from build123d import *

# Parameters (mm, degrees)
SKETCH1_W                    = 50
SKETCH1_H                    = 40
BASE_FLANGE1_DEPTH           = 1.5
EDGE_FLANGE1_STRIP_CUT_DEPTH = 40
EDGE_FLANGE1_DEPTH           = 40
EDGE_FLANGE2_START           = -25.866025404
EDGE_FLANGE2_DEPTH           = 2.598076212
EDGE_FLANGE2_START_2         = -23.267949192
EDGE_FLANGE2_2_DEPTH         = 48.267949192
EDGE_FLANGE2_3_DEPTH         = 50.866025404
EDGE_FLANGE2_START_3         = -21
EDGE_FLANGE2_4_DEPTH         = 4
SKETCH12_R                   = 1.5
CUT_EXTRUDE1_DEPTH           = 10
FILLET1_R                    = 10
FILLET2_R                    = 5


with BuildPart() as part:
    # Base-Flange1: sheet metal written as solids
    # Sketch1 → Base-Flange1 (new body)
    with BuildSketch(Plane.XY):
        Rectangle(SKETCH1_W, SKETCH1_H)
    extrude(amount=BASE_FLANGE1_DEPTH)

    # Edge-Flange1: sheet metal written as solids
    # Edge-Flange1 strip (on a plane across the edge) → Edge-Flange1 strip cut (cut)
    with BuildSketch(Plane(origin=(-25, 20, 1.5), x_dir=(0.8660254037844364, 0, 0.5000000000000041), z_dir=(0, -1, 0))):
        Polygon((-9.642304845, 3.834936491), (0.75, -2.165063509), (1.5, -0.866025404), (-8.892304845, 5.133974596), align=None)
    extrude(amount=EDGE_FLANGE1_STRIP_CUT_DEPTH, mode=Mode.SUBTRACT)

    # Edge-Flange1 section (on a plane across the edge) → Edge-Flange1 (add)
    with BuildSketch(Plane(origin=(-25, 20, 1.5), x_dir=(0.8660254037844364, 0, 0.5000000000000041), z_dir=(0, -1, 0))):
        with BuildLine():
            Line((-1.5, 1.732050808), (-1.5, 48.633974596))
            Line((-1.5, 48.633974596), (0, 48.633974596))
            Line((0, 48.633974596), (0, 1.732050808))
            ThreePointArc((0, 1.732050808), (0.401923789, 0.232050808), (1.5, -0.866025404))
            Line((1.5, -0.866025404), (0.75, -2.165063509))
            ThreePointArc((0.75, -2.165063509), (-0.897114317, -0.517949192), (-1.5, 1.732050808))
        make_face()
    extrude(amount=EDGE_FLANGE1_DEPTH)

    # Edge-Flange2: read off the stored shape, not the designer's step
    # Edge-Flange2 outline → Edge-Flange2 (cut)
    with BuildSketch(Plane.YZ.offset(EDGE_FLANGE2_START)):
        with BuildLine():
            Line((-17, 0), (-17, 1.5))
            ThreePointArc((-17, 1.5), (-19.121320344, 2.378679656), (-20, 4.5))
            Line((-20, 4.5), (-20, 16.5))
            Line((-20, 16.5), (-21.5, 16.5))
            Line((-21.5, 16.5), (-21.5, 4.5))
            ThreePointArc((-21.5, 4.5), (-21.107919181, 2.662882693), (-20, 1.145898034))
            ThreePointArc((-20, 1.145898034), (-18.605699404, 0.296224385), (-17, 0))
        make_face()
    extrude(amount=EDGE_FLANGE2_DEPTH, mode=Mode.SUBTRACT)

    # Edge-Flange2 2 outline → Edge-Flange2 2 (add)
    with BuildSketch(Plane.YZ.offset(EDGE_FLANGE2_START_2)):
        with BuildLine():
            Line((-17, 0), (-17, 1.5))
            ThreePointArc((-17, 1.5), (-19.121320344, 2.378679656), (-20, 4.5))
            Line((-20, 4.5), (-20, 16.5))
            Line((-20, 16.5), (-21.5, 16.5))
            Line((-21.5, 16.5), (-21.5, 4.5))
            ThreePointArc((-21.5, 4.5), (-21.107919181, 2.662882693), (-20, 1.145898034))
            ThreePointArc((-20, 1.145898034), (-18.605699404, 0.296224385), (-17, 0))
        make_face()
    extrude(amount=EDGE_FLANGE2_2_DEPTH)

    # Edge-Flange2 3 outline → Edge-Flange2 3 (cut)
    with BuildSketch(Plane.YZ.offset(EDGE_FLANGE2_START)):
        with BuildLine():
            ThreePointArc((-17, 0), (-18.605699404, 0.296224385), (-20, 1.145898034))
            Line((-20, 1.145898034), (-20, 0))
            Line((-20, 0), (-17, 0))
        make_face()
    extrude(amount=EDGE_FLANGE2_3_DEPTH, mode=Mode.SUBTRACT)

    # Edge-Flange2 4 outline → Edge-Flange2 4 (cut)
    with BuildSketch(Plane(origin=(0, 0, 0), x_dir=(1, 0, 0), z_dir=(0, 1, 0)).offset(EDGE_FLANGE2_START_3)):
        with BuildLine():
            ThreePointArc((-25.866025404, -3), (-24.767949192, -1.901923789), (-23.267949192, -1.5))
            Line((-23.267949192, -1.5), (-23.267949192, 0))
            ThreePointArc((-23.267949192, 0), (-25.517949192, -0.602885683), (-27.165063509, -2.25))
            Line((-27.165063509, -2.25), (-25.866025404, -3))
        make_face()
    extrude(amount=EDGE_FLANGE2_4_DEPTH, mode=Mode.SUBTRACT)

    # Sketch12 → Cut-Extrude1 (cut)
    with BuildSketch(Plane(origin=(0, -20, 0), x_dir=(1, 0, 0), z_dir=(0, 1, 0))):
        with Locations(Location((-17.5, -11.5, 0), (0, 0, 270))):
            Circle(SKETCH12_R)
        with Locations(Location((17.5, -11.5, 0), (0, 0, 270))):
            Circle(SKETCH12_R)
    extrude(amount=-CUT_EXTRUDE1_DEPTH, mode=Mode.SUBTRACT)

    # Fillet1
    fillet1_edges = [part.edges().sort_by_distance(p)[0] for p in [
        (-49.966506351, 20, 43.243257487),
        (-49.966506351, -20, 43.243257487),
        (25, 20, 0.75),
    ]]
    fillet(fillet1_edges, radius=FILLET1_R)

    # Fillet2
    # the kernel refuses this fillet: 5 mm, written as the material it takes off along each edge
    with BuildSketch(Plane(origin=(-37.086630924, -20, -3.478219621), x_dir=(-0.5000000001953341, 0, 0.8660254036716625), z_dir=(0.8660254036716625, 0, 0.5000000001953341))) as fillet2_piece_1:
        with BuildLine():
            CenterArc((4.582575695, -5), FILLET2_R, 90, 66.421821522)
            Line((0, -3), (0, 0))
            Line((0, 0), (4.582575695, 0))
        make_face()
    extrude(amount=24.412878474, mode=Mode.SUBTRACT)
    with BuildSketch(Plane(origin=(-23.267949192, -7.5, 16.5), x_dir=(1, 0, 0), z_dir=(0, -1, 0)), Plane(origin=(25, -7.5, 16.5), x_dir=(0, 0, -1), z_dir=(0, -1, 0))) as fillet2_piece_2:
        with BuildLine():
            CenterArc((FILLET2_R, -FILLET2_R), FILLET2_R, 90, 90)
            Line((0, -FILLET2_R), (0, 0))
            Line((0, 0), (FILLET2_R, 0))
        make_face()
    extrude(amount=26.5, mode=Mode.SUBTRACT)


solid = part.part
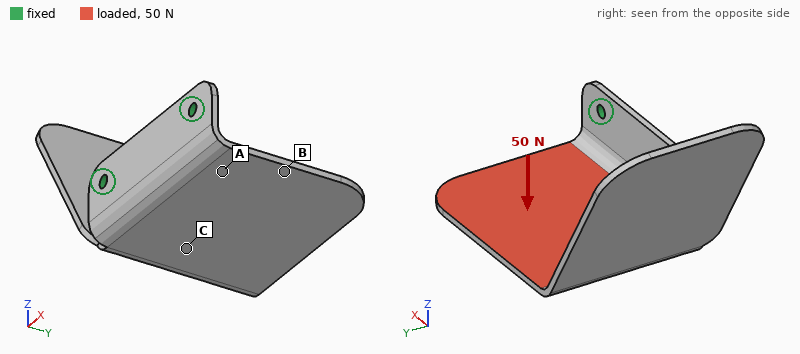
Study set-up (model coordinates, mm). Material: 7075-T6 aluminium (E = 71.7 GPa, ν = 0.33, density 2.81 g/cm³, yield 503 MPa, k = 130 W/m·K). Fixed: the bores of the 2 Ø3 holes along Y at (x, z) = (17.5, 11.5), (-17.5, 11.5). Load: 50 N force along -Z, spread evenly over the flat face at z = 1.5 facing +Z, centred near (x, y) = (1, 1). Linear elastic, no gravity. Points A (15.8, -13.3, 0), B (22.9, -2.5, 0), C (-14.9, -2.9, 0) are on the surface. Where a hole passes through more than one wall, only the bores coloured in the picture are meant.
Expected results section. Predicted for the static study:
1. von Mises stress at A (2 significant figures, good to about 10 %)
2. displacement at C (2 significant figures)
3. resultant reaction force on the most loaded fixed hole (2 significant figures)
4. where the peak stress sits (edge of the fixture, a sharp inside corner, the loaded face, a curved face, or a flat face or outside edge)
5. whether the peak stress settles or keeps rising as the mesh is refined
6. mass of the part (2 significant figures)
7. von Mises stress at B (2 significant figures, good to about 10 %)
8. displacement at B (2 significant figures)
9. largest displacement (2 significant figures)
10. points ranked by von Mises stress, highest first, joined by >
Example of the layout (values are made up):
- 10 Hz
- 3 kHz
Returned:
- 33 MPa
- 0.34 mm
- 29 N
- edge of the fixture
- keeps rising
- 19 g
- 16 MPa
- 0.32 mm
- 1.1 mm
- A > B > C
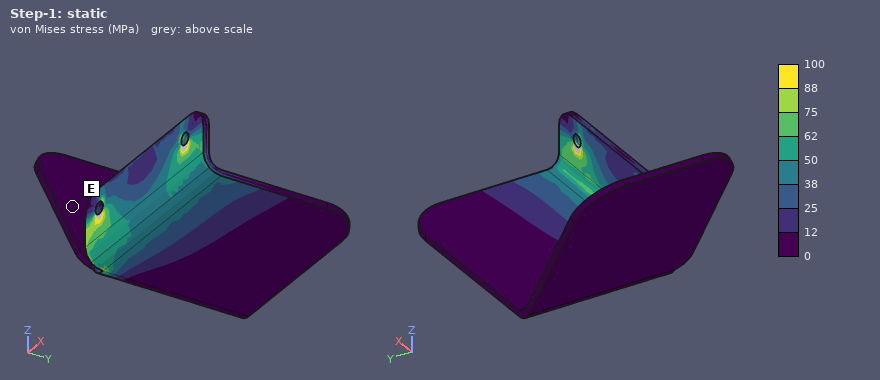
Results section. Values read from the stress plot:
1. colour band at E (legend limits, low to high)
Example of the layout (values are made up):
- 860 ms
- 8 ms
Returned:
- 0 to 12 MPa
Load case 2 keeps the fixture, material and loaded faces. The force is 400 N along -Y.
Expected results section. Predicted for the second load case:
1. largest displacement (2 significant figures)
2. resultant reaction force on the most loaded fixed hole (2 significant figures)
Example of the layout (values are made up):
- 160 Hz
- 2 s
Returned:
- 1.1 mm
- 210 N
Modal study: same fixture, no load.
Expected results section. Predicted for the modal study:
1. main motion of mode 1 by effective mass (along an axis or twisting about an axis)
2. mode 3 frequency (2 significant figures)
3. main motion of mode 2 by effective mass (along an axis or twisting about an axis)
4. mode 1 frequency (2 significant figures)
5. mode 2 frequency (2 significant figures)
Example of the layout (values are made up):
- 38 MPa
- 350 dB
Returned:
- along Z
- 1000 Hz
- along X
- 250 Hz
- 400 Hz
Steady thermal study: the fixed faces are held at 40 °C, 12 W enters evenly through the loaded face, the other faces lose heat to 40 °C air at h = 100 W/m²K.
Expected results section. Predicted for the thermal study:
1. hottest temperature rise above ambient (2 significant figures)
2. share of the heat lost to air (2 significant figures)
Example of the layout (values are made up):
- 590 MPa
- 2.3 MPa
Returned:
- 22 K
- 58 %
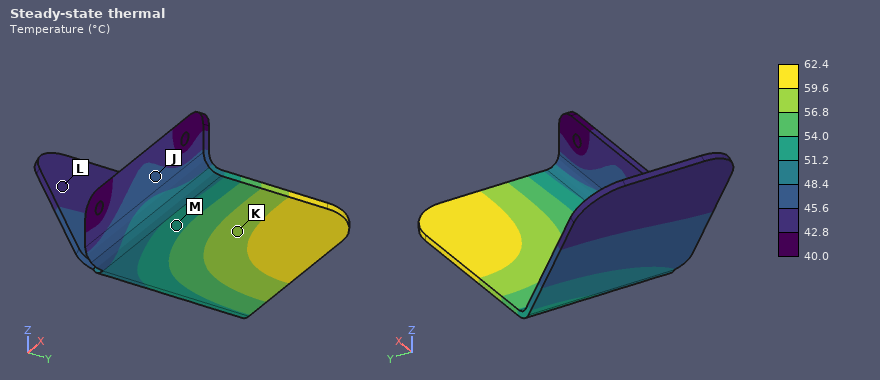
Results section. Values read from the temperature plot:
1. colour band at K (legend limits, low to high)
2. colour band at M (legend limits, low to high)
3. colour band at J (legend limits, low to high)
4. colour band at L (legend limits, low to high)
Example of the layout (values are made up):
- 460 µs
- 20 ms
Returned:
- 56.8 to 59.6 °C
- 51.2 to 54.0 °C
- 45.6 to 48.4 °C
- 42.8 to 45.6 °C
